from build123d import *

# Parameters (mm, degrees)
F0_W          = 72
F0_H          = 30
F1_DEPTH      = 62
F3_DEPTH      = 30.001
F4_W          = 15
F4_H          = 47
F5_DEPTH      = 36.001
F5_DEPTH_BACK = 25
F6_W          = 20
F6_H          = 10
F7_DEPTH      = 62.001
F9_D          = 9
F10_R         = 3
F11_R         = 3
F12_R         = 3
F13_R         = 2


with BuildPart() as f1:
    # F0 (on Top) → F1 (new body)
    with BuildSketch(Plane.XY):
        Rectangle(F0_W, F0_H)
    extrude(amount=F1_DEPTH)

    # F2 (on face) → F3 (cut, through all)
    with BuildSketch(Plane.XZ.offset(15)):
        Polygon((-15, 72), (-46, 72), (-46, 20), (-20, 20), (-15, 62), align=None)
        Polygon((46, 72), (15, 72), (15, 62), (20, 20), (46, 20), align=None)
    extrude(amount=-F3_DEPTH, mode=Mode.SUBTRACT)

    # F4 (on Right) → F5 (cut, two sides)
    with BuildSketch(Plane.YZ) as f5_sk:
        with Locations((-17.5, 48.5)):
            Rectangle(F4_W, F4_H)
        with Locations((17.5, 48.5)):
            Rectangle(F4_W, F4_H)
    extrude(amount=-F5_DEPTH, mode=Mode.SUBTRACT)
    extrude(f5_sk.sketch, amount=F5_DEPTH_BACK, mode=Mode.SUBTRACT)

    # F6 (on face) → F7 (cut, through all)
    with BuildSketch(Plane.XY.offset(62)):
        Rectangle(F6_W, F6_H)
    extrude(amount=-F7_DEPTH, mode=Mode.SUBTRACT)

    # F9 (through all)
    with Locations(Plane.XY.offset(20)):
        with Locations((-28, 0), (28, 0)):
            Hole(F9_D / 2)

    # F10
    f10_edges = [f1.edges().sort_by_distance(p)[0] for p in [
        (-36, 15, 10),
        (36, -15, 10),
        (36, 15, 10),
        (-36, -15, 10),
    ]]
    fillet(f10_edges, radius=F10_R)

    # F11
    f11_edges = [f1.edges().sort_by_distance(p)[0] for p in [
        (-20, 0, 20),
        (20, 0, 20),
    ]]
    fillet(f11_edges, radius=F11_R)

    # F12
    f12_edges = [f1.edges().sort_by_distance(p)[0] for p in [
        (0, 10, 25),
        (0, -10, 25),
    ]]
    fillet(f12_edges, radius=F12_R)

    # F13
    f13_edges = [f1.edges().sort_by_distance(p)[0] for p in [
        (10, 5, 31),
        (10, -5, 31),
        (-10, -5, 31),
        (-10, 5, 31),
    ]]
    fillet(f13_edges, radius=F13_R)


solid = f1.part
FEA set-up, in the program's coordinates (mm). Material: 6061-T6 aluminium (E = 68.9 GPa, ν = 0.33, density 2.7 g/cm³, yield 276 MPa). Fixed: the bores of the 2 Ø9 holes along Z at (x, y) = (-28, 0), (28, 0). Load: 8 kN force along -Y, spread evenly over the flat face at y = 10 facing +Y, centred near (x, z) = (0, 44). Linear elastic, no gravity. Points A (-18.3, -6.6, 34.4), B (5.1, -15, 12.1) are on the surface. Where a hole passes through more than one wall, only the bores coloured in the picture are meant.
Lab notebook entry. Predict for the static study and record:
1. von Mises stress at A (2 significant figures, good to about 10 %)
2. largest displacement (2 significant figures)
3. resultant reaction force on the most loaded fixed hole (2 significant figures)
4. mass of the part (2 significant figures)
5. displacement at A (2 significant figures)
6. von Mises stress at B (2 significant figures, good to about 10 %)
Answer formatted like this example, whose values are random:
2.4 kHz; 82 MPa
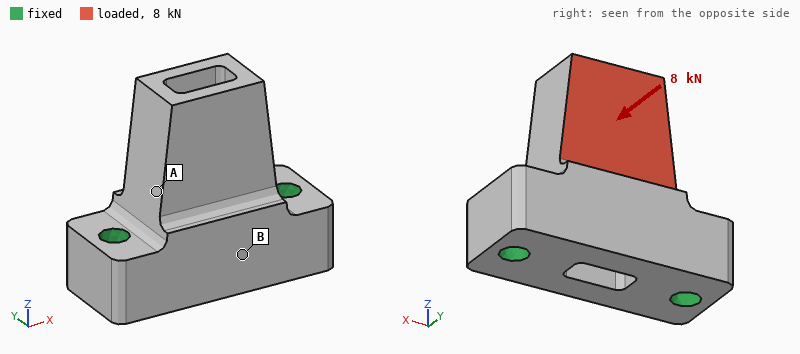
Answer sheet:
42 MPa; 0.17 mm; 4.0 kN; 160 g; 0.056 mm; 20 MPa
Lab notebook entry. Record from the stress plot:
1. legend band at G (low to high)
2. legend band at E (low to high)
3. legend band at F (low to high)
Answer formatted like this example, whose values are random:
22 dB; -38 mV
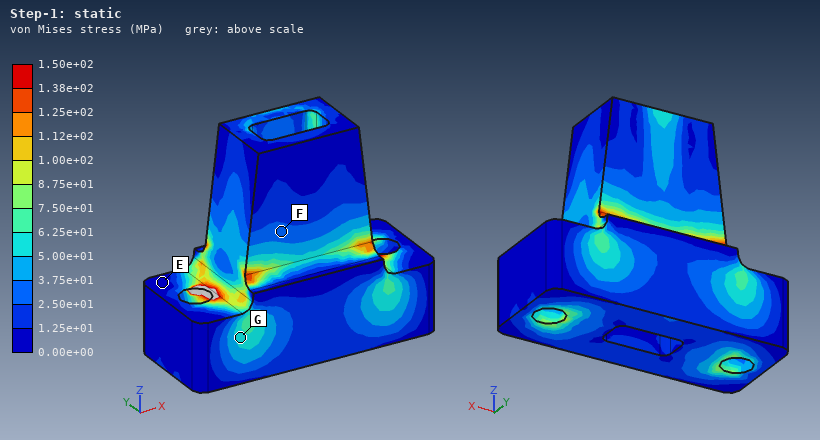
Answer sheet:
5.00e+01 to 6.25e+01 MPa; 0.00e+00 to 1.25e+01 MPa; 2.50e+01 to 3.75e+01 MPa
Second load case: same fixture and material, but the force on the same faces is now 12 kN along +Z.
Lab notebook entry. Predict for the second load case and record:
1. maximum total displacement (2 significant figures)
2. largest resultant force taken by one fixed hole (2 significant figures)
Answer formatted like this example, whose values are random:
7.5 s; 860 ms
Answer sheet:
0.11 mm; 6.3 kN
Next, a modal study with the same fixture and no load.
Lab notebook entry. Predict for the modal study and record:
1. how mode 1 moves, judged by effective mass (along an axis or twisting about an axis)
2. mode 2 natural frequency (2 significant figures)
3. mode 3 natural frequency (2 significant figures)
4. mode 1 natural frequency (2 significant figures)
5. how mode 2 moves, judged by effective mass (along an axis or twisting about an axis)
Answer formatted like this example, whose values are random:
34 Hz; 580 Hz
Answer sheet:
along Y; 12 kHz; 16 kHz; 6300 Hz; along X
